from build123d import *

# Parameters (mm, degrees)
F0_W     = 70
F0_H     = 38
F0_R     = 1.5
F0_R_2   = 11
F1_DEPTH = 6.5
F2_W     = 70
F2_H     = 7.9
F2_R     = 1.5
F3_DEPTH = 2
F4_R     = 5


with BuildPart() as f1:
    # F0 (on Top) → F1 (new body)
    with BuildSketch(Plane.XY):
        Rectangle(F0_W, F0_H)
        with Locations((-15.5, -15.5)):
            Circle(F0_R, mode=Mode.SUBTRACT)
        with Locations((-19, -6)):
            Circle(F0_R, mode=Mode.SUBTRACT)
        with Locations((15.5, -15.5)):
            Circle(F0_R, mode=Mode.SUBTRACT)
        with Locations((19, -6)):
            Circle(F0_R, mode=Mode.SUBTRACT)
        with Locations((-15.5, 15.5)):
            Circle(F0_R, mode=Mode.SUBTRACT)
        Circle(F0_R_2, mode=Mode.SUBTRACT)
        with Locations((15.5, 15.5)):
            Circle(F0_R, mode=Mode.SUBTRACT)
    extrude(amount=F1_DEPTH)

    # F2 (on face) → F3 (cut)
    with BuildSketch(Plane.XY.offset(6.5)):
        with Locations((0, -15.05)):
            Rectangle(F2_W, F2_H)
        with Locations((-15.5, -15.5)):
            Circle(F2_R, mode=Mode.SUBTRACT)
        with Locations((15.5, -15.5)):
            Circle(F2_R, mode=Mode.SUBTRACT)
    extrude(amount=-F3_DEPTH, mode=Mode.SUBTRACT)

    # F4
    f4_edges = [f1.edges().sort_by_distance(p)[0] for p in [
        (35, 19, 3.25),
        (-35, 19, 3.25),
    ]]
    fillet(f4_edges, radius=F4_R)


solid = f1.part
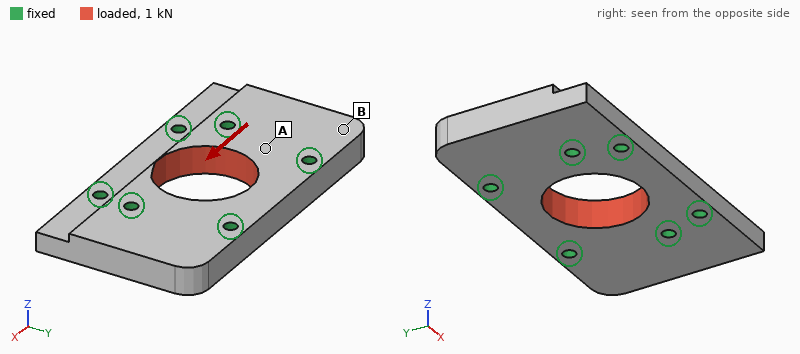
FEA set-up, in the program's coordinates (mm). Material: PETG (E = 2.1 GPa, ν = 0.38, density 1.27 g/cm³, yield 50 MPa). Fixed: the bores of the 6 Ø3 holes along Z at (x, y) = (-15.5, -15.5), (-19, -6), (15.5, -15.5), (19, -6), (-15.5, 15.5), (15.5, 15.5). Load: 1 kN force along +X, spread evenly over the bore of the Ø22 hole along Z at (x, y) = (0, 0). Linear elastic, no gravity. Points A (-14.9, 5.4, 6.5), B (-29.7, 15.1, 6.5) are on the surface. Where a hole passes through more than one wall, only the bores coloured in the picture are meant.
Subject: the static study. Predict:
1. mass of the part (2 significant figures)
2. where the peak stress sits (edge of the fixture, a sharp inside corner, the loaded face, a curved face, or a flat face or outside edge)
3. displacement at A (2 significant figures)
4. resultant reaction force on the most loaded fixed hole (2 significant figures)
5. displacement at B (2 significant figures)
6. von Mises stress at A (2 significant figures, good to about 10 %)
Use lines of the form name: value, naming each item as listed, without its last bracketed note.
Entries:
mass of the part: 17 g
where the peak stress sits: a flat face or outside edge
displacement at A: 14 µm
resultant reaction force on the most loaded fixed hole: 220 N
displacement at B: 5.4 µm
von Mises stress at A: 1.5 MPa
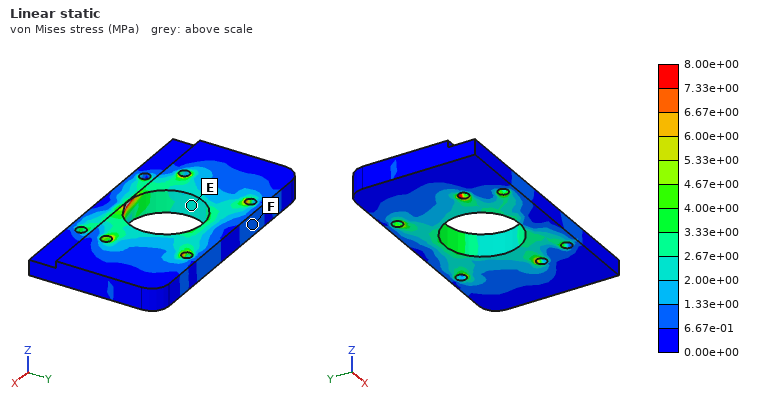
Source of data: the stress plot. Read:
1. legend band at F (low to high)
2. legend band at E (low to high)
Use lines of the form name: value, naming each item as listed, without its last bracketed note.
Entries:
legend band at F: 6.67e-01 to 1.33e+00 MPa
legend band at E: 2.00e+00 to 2.67e+00 MPa
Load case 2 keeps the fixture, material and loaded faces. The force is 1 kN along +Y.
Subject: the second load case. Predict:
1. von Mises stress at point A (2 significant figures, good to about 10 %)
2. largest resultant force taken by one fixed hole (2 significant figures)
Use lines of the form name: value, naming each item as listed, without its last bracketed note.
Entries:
von Mises stress at point A: 3.2 MPa
largest resultant force taken by one fixed hole: 220 N
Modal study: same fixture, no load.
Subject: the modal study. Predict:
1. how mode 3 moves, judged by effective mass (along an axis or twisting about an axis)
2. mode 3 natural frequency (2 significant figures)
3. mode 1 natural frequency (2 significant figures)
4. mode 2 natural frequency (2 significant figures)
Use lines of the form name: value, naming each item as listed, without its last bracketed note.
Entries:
how mode 3 moves, judged by effective mass: twisting about X
mode 3 natural frequency: 5000 Hz
mode 1 natural frequency: 3600 Hz
mode 2 natural frequency: 3600 Hz
